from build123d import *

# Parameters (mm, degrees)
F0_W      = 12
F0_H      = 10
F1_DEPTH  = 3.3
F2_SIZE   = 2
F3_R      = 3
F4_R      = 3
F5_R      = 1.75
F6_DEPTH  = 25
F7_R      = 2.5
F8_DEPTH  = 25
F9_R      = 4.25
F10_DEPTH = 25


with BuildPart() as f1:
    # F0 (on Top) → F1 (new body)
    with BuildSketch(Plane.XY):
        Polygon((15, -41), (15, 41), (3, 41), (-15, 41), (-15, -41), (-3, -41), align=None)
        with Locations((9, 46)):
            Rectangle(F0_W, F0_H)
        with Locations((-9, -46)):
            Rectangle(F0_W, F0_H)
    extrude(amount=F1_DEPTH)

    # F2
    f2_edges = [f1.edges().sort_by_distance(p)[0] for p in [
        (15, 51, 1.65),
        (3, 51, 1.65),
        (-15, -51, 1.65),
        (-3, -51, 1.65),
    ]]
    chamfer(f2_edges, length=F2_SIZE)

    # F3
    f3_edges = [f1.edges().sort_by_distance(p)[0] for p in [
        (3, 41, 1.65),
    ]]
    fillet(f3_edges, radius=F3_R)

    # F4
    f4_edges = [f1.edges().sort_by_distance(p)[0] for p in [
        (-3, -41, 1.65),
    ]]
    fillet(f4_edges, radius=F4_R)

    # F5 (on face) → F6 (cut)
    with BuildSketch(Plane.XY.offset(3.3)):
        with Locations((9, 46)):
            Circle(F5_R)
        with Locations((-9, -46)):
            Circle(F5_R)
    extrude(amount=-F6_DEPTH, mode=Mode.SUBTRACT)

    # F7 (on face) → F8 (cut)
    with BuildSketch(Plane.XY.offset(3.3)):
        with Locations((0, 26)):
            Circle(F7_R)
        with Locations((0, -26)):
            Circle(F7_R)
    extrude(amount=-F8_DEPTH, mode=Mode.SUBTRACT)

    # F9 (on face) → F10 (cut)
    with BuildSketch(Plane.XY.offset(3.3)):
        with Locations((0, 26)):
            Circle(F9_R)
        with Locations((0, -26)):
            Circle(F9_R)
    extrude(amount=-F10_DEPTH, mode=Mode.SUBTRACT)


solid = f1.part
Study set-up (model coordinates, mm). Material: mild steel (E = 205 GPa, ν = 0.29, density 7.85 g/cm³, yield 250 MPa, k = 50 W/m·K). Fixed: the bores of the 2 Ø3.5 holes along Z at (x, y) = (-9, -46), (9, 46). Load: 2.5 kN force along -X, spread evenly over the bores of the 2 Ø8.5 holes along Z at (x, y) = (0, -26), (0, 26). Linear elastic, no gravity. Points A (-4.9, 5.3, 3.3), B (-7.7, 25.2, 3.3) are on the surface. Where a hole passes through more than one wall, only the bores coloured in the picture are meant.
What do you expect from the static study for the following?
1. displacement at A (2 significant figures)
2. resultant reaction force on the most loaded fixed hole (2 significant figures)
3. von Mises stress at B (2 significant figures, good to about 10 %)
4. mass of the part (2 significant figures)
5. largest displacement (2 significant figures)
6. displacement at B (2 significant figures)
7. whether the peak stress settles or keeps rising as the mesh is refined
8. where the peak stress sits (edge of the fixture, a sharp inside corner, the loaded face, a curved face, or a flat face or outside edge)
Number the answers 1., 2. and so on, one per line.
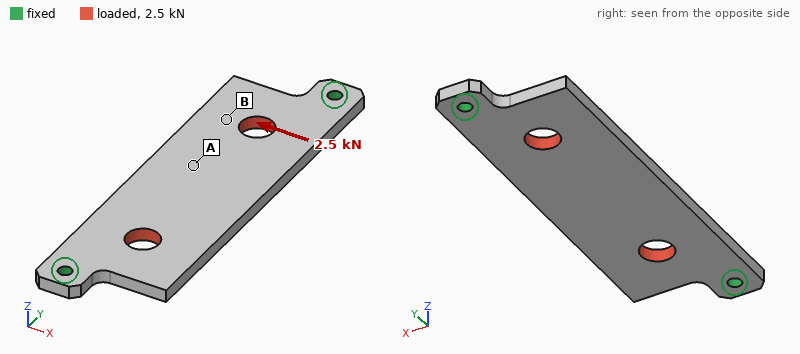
1. 20 µm
2. 1.3 kN
3. 36 MPa
4. 66 g
5. 20 µm
6. 16 µm
7. keeps rising
8. edge of the fixture
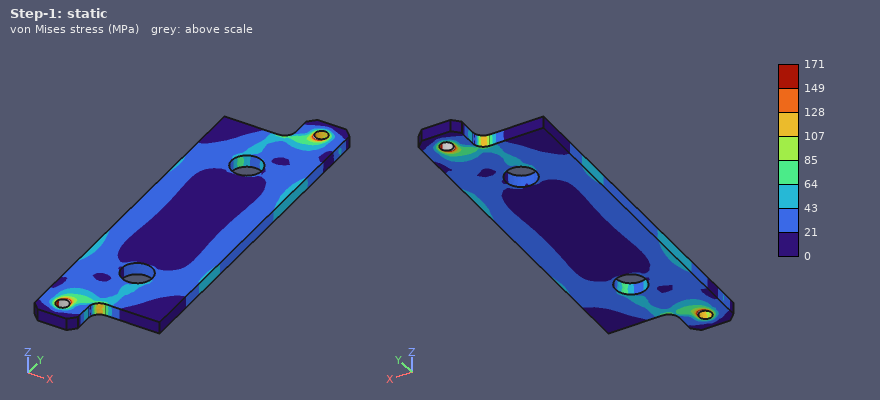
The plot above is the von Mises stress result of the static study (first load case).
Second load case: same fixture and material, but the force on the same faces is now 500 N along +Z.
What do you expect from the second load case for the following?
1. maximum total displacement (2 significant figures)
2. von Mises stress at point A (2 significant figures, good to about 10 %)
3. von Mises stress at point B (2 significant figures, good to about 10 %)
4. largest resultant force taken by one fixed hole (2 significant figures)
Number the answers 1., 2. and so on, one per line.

1. 82 µm
2. 31 MPa
3. 42 MPa
4. 250 N
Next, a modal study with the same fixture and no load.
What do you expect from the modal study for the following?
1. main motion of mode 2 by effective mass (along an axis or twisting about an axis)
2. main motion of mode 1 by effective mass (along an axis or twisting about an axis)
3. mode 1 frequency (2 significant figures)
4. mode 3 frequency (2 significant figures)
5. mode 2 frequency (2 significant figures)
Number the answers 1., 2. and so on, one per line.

1. twisting about Y
2. along Z
3. 1600 Hz
4. 4900 Hz
5. 2400 Hz
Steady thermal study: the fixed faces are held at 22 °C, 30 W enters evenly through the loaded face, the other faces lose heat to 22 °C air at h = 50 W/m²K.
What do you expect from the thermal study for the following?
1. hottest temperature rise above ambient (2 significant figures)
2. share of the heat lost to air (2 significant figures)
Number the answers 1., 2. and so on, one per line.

1. 72 K
2. 48 %
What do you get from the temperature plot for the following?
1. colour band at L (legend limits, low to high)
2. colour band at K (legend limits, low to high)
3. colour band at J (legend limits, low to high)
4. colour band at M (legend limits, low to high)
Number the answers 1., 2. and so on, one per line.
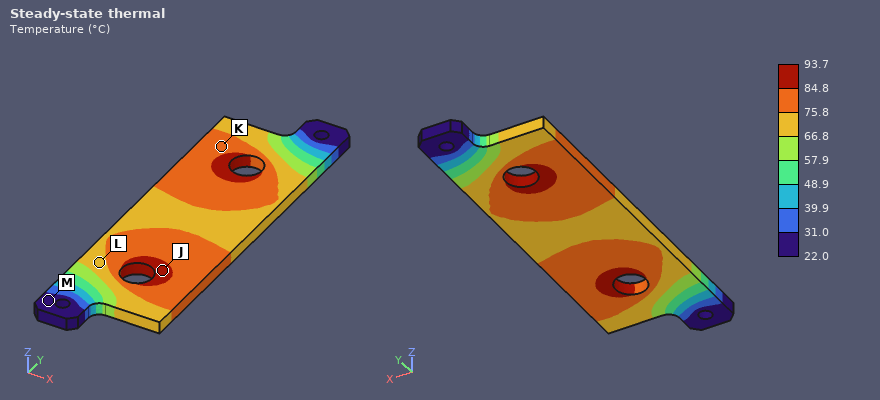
1. 66.8 to 75.8 °C
2. 75.8 to 84.8 °C
3. 84.8 to 93.7 °C
4. 22.0 to 31.0 °C
